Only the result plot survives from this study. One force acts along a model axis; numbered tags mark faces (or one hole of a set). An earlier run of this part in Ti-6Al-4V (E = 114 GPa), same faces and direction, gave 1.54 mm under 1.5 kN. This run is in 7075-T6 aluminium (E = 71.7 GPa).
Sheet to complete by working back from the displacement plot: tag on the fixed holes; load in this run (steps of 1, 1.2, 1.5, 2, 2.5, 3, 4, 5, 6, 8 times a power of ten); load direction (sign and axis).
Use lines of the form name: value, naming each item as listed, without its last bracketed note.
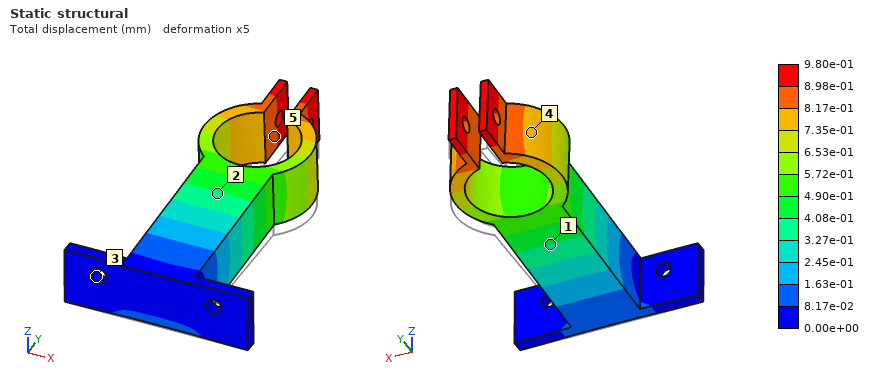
tag on the fixed holes: 3
load in this run: 600 N
load direction: +Z
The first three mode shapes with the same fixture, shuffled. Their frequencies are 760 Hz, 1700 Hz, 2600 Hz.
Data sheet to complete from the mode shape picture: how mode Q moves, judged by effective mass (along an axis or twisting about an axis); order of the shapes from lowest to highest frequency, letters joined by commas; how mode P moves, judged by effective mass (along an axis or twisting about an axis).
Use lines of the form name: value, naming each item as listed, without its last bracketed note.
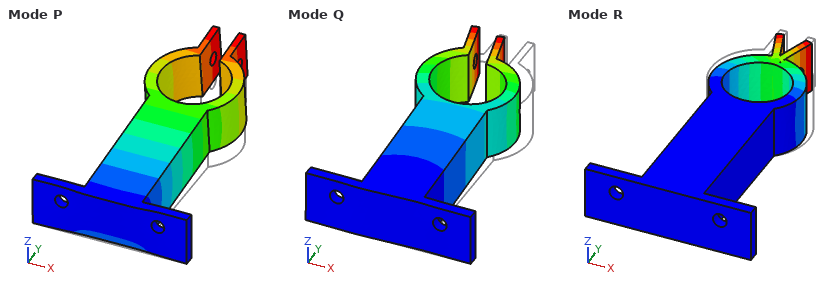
how mode Q moves, judged by effective mass: along X
order of the shapes from lowest to highest frequency, letters joined by commas: P, Q, R
how mode P moves, judged by effective mass: along Z
